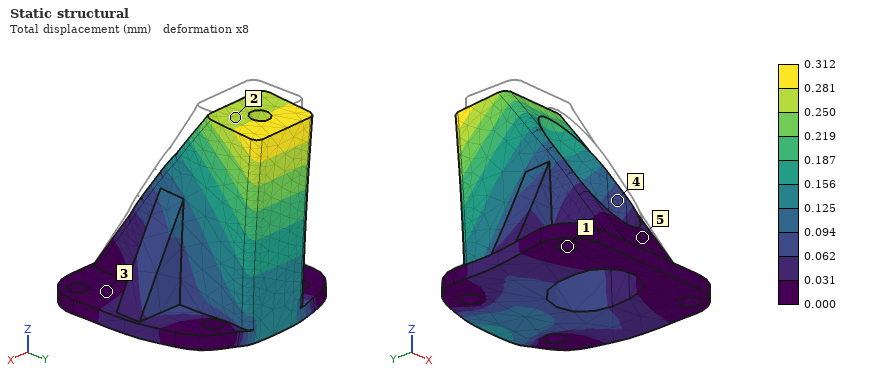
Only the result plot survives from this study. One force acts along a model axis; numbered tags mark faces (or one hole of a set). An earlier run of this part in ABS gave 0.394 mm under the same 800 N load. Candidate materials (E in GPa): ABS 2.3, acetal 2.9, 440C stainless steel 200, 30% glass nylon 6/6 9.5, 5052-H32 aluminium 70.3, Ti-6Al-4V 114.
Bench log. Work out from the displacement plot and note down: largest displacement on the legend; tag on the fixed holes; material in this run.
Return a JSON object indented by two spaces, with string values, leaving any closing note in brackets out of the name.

{
  "largest displacement on the legend": "0.312 mm",
  "tag on the fixed holes": "1",
  "material in this run": "acetal"
}
